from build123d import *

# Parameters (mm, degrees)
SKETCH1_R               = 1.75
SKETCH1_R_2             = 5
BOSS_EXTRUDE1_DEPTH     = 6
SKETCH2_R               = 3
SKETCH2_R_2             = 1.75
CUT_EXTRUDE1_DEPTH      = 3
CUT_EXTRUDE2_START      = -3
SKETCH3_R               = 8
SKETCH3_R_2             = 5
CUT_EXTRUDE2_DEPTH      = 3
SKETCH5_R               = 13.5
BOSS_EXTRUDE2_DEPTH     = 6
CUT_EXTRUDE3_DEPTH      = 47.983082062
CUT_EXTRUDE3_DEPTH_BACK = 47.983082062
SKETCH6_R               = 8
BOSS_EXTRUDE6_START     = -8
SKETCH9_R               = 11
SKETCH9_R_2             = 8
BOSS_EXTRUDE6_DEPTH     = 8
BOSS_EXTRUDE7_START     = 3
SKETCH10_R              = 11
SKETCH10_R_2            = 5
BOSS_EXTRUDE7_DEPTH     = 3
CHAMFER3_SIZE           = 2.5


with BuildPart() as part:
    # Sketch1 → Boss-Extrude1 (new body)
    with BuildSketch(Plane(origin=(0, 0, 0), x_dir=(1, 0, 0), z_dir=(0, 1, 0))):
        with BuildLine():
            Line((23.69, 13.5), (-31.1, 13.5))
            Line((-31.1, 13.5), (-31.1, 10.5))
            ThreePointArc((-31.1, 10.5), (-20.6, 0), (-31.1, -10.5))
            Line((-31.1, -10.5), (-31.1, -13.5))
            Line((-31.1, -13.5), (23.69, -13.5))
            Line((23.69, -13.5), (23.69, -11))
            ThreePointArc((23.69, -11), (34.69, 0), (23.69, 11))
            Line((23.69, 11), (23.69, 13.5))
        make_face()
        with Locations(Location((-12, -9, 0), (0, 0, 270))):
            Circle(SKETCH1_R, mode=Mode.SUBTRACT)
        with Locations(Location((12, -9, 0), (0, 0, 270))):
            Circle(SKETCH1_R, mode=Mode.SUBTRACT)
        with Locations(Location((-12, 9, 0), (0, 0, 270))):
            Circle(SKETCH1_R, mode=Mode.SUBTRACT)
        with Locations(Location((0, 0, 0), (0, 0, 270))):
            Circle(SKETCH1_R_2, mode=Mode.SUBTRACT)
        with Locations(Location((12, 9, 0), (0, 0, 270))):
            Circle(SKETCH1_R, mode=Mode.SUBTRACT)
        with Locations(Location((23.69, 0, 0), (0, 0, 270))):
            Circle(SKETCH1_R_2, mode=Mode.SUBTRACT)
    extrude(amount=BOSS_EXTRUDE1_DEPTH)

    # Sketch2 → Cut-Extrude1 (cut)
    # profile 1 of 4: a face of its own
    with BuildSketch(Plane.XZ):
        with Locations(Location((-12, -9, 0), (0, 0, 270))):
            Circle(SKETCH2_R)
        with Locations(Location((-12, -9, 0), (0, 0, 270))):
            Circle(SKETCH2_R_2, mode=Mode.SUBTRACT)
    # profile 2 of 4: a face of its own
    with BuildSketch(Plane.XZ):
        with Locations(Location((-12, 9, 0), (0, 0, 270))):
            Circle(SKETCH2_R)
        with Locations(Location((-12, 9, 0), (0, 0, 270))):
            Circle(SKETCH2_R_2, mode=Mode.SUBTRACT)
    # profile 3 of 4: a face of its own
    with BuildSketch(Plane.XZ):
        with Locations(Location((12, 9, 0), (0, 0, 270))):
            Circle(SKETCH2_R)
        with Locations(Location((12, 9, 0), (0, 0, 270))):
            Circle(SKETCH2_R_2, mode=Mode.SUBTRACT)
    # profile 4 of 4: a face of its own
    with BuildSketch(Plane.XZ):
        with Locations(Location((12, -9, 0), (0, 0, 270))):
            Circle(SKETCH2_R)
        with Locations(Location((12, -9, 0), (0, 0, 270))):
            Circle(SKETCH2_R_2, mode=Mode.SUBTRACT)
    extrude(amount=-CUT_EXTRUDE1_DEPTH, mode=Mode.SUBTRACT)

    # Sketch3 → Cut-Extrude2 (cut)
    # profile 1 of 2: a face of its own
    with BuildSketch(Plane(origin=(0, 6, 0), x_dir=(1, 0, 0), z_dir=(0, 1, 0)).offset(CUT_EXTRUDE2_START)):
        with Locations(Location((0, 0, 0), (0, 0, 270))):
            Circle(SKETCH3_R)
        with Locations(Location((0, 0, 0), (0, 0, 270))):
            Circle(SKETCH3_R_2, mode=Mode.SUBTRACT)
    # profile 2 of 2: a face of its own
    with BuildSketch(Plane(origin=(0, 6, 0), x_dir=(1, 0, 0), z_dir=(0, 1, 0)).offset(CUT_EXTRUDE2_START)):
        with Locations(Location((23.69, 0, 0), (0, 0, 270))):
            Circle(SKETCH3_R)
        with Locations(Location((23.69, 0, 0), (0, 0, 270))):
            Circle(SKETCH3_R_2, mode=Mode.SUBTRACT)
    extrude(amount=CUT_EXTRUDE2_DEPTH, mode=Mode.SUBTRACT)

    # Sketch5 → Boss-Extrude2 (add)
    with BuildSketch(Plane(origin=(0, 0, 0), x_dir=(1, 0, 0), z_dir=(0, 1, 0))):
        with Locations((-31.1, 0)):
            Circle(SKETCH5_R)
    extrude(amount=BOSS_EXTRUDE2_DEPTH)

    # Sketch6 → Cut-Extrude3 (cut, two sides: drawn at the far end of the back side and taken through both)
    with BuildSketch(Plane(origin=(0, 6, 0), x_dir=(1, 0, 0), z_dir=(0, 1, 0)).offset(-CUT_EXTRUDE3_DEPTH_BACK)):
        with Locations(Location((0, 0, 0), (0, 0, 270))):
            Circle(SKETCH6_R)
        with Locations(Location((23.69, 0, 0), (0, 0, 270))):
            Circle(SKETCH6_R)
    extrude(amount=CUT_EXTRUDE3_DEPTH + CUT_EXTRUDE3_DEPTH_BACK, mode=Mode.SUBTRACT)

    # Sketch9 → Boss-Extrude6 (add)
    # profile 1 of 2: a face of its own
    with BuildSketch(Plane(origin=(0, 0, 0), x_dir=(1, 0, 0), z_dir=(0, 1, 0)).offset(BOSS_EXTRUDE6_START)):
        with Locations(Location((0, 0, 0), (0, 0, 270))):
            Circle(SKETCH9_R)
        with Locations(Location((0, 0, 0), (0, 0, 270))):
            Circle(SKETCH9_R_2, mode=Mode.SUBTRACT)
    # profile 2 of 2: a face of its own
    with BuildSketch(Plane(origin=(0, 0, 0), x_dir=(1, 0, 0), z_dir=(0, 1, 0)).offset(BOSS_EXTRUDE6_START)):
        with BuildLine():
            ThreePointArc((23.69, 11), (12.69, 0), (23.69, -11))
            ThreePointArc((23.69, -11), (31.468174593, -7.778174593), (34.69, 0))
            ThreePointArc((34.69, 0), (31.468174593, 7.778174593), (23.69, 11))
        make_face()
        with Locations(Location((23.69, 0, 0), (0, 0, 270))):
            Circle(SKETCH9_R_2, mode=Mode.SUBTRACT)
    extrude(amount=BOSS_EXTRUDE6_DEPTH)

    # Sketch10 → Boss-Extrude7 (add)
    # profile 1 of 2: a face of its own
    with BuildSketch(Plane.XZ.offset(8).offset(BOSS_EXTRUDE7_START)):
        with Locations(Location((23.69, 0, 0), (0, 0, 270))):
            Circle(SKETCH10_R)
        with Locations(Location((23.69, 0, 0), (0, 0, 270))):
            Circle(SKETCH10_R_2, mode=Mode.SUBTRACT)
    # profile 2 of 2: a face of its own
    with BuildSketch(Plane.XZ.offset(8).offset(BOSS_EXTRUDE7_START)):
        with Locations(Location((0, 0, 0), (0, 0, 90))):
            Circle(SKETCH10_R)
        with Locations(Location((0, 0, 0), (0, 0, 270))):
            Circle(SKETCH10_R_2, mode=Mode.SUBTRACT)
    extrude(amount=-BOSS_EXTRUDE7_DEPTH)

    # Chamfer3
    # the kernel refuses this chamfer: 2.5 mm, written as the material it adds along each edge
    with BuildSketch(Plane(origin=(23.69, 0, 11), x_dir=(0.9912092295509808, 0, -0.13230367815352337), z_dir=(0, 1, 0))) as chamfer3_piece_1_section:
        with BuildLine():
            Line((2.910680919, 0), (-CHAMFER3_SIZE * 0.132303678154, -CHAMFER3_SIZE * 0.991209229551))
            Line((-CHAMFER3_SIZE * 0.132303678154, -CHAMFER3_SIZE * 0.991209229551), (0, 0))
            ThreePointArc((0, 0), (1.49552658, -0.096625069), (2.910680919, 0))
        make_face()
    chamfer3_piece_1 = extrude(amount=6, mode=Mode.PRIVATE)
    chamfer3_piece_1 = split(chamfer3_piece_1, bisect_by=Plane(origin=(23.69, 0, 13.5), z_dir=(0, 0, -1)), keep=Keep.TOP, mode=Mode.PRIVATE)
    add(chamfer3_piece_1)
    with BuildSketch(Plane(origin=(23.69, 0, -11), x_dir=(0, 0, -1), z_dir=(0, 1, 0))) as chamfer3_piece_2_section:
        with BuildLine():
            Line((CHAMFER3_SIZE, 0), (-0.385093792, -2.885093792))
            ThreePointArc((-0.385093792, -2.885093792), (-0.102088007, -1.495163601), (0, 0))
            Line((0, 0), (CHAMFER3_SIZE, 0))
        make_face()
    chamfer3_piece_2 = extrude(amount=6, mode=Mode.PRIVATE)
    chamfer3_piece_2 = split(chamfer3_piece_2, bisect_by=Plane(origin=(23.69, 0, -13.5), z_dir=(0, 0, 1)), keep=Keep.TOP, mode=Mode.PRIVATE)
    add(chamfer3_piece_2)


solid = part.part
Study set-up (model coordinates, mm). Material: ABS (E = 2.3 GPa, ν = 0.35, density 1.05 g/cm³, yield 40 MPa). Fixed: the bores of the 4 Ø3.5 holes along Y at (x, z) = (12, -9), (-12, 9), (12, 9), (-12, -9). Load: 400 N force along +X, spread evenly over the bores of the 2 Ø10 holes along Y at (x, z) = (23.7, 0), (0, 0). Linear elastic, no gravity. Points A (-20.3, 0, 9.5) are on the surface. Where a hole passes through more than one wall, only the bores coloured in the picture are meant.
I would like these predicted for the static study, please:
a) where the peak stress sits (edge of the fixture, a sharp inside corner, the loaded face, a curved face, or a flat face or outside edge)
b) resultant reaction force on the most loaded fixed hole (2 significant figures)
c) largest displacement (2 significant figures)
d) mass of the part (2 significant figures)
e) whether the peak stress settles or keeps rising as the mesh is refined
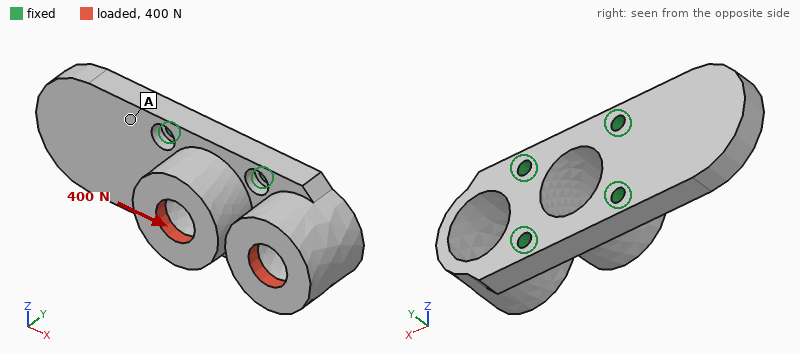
edge of the fixture
140 N
0.79 mm
14 g
keeps rising
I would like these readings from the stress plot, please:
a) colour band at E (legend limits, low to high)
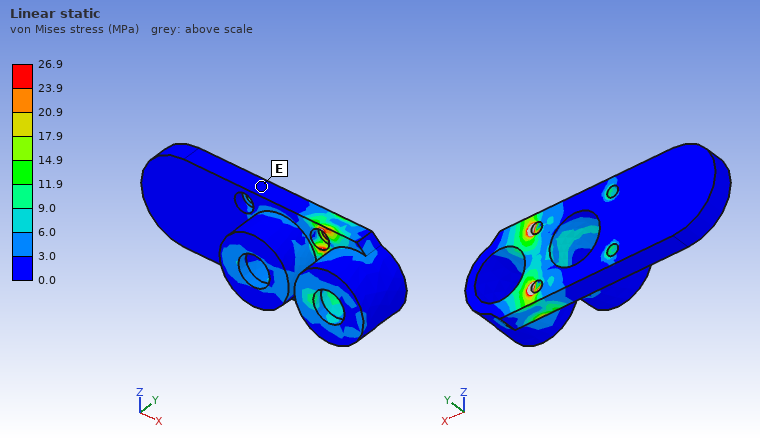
0.0 to 3.0 MPa
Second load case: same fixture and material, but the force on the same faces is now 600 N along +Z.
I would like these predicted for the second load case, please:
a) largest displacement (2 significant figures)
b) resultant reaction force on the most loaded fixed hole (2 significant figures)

0.26 mm
420 N
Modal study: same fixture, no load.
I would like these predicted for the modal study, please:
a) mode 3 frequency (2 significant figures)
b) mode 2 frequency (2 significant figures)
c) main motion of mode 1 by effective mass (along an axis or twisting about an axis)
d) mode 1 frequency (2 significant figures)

3700 Hz
1700 Hz
along Y
1200 Hz
